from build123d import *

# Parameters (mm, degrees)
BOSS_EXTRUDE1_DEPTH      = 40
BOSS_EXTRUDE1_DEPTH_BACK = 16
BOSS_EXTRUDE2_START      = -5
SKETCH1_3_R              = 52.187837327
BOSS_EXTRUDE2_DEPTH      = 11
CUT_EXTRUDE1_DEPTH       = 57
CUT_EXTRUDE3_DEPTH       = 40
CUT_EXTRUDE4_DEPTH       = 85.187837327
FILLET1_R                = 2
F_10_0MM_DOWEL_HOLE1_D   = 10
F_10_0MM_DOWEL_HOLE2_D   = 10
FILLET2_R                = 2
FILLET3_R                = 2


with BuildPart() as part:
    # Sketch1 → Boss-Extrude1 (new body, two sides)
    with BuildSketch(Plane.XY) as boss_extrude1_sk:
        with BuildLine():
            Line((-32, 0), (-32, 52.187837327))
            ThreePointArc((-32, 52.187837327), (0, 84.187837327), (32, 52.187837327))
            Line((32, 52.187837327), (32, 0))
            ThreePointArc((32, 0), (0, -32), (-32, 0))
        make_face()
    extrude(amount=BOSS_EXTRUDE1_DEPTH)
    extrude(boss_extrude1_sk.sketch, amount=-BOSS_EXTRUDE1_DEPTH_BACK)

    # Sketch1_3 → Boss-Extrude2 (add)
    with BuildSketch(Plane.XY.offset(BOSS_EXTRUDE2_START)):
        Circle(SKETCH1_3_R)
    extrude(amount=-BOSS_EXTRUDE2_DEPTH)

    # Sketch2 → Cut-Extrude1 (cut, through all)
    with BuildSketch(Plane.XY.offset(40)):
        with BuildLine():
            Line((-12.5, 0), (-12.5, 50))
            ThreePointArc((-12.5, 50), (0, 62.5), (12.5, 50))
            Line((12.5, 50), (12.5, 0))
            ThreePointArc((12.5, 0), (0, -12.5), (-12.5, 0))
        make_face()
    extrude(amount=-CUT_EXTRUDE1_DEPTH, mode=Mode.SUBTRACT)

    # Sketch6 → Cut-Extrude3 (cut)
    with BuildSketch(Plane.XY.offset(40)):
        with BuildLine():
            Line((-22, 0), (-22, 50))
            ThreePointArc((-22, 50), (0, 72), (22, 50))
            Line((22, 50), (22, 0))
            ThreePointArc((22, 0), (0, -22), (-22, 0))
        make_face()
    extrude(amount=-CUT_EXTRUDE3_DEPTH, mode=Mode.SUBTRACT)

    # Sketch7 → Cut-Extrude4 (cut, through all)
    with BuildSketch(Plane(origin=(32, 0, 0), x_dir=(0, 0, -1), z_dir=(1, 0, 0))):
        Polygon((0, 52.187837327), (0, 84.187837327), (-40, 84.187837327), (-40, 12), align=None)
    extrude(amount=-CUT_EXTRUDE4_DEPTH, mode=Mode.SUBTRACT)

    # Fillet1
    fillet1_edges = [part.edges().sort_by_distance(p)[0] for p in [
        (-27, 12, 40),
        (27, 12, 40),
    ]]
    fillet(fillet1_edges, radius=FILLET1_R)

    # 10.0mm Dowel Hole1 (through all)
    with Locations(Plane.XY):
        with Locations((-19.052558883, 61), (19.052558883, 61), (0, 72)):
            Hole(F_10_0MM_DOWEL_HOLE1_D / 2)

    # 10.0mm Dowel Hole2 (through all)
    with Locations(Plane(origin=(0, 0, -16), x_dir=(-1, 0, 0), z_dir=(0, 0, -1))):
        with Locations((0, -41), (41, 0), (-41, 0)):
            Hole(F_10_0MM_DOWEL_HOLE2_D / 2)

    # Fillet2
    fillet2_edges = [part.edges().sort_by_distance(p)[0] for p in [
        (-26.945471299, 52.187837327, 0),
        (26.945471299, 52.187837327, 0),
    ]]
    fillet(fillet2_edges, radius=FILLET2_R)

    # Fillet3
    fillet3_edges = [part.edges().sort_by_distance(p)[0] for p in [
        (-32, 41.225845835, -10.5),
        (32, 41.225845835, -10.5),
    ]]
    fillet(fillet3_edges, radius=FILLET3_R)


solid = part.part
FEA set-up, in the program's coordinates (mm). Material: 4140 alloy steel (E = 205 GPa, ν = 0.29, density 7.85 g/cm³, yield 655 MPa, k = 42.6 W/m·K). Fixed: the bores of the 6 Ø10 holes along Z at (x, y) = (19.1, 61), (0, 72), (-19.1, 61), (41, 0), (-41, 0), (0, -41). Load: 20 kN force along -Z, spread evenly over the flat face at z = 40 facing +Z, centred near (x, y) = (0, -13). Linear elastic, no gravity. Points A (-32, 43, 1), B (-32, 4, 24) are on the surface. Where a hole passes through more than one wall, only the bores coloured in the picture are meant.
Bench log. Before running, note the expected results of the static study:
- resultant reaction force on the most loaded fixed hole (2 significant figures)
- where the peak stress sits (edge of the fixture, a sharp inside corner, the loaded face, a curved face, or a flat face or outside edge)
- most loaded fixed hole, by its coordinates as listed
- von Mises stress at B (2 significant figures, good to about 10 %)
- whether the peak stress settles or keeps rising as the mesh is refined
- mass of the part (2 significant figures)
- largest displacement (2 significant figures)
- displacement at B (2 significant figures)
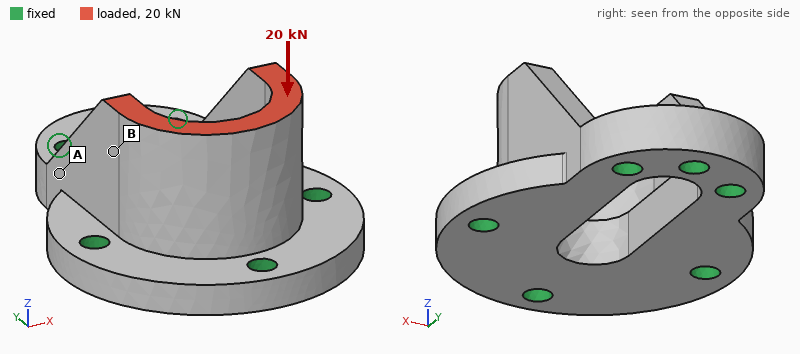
8.6 kN
edge of the fixture
(0, -41)
16 MPa
keeps rising
1.4 kg
12 µm
6.1 µm
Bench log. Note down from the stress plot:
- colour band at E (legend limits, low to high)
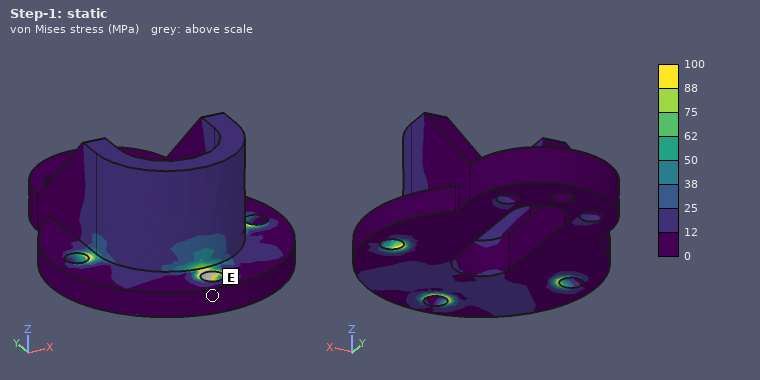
0 to 12 MPa
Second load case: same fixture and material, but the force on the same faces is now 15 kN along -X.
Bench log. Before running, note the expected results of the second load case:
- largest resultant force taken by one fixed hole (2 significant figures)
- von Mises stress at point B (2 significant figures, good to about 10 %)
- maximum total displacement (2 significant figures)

12 kN
60 MPa
69 µm
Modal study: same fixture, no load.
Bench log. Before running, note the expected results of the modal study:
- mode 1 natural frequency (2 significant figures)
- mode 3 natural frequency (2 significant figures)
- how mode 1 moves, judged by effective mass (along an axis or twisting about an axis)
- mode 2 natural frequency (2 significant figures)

6400 Hz
9900 Hz
along X
7100 Hz
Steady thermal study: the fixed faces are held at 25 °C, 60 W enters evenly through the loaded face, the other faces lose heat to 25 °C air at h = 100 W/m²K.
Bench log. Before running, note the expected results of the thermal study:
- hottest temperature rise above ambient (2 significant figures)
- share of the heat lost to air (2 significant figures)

47 K
53 %
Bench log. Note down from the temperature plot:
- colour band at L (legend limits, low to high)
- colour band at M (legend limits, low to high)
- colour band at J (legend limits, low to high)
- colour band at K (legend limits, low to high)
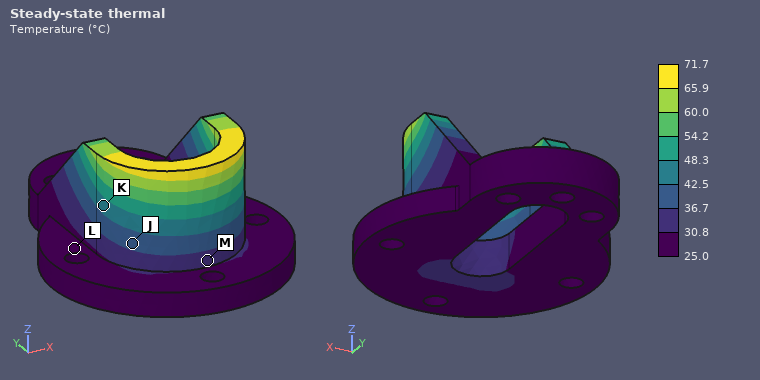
25.0 to 30.8 °C
30.8 to 36.7 °C
36.7 to 42.5 °C
42.5 to 48.3 °C
